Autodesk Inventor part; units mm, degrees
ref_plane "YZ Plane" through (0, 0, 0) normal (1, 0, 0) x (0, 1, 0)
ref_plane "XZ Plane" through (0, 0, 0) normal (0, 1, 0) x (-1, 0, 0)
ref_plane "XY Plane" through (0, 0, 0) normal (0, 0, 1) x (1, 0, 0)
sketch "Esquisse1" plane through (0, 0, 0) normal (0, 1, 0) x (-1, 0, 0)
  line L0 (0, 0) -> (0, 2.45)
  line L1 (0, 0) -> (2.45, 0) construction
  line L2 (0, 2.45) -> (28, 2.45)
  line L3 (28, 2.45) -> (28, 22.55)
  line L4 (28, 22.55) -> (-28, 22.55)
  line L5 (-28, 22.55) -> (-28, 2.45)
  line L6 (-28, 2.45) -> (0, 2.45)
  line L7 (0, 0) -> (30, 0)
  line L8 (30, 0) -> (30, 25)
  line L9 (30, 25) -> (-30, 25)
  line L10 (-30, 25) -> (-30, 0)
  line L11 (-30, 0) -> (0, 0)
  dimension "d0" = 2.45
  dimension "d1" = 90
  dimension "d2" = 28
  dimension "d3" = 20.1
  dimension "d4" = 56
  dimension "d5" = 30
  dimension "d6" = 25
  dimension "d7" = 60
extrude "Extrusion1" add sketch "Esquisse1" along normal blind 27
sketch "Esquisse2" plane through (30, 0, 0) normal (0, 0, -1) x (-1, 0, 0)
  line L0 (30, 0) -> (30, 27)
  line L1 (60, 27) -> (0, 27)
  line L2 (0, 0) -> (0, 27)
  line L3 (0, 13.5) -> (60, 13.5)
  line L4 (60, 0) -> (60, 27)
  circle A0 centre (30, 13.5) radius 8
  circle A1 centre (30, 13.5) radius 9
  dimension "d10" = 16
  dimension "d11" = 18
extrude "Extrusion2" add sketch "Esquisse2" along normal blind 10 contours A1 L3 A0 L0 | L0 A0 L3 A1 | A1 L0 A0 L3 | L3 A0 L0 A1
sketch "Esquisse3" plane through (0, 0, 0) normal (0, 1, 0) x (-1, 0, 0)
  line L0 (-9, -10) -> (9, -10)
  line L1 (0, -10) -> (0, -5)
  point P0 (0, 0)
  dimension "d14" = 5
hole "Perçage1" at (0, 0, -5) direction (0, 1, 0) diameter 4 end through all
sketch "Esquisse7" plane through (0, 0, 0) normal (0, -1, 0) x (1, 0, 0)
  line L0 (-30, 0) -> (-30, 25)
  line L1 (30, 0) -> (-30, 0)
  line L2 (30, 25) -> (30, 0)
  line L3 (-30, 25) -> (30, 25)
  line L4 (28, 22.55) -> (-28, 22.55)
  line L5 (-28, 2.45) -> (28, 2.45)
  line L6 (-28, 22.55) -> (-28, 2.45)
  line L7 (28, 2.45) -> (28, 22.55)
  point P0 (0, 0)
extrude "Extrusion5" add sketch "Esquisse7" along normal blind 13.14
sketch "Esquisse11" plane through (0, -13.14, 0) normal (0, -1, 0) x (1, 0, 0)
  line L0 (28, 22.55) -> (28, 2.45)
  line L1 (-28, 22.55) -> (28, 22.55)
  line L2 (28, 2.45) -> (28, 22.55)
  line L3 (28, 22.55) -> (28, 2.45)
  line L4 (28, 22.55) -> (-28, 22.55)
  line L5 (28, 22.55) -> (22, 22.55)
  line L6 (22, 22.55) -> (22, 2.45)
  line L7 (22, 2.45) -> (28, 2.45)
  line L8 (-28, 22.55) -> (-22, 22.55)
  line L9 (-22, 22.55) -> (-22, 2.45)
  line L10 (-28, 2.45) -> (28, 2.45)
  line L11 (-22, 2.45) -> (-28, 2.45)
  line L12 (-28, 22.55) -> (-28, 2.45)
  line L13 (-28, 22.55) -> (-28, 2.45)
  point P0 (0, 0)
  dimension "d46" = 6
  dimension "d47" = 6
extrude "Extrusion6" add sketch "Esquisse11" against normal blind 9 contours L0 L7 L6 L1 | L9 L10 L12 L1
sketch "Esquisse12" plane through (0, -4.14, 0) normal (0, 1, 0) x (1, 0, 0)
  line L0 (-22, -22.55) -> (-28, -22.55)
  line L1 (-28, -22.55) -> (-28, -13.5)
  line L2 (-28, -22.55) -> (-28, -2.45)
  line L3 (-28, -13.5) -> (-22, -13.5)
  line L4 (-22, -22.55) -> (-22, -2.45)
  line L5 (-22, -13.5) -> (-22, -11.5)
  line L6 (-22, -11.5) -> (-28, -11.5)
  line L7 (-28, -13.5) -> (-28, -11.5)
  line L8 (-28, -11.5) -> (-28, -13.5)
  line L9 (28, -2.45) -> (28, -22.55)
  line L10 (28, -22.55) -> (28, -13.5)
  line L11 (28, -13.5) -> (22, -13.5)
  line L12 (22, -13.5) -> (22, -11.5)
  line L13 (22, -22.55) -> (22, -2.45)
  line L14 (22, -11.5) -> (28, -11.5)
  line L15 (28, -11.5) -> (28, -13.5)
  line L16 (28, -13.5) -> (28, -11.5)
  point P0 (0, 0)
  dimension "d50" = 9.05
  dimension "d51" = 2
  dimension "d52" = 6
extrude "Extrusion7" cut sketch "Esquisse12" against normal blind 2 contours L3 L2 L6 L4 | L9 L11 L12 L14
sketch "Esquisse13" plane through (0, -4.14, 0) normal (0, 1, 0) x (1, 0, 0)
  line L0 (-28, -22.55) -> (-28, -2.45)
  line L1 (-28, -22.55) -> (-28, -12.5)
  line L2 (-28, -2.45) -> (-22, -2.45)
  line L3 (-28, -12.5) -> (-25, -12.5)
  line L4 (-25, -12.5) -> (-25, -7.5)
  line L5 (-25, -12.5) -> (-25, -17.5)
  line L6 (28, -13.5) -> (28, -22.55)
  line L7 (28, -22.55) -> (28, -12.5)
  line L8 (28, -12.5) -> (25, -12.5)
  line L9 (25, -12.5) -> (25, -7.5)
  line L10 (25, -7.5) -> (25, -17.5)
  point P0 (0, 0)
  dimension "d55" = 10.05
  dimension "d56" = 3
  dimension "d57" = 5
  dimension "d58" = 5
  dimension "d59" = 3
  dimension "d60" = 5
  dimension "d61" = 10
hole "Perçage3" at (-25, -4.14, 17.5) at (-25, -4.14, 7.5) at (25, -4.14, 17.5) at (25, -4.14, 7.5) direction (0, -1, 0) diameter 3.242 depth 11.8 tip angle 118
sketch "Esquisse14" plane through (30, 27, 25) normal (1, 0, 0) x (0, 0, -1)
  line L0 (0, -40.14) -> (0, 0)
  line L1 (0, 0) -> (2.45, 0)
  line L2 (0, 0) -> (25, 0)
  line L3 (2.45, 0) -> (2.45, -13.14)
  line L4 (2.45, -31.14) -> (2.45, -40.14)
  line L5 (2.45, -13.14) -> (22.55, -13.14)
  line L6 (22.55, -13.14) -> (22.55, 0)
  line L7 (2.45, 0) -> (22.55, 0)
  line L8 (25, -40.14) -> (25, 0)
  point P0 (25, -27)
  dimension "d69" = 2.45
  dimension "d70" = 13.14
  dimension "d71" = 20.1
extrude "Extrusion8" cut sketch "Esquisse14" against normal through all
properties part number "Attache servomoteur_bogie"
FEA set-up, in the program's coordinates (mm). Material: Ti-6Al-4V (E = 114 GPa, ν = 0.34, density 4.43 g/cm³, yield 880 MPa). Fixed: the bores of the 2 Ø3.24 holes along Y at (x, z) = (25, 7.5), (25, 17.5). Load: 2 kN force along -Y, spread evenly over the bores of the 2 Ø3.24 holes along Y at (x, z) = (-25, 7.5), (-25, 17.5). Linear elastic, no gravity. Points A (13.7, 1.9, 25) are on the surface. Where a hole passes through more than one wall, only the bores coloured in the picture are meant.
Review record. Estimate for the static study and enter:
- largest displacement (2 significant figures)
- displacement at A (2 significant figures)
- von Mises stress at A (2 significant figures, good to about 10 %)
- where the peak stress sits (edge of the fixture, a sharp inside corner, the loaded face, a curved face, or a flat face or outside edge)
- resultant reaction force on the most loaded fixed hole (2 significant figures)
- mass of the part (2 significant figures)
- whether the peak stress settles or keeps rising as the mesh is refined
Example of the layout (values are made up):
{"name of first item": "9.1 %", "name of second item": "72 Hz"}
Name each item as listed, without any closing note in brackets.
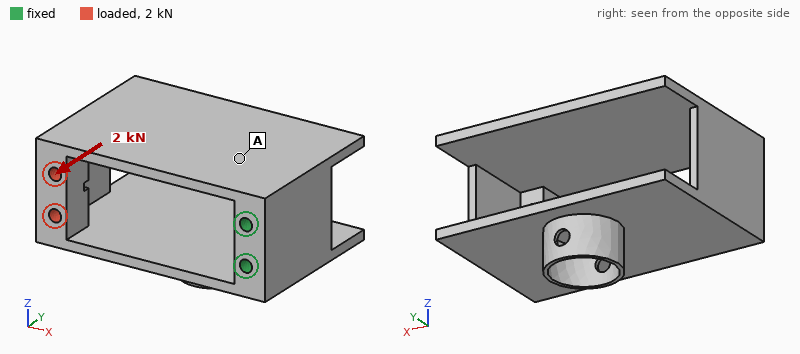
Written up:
{"largest displacement": "0.79 mm", "displacement at A": "0.18 mm", "von Mises stress at A": "67 MPa", "where the peak stress sits": "edge of the fixture", "resultant reaction force on the most loaded fixed hole": "1.0 kN", "mass of the part": "72 g", "whether the peak stress settles or keeps rising as the mesh is refined": "keeps rising"}
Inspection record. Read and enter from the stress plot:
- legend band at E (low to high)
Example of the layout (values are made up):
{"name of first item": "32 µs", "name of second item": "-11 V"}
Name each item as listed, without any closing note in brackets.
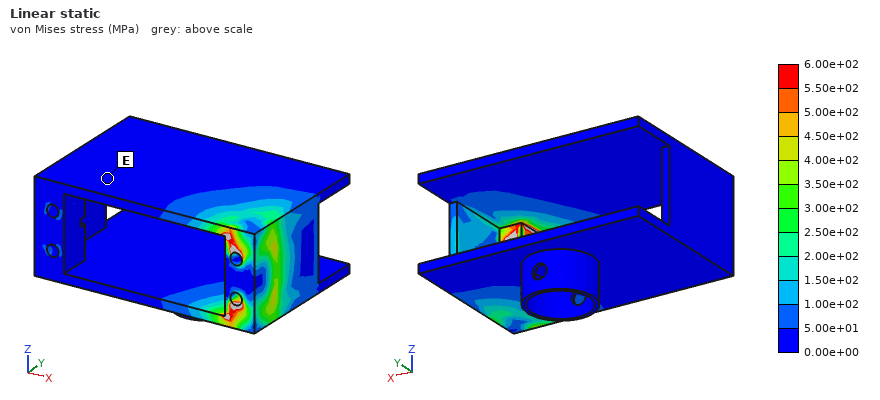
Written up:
{"legend band at E": "0.00e+00 to 5.00e+01 MPa"}
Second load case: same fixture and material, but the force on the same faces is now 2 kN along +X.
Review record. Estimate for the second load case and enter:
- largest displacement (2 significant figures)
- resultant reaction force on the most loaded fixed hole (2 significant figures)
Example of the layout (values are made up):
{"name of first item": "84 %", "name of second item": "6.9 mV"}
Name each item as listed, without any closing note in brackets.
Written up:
{"largest displacement": "41 µm", "resultant reaction force on the most loaded fixed hole": "1.1 kN"}
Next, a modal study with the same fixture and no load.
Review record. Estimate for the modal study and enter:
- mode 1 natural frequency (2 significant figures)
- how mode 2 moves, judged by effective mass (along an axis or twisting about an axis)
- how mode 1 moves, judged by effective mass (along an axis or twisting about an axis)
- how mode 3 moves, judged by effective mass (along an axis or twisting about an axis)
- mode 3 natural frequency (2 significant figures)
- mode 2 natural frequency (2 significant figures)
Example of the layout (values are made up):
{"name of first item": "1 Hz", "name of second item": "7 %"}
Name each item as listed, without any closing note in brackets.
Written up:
{"mode 1 natural frequency": "770 Hz", "how mode 2 moves, judged by effective mass": "along Y", "how mode 1 moves, judged by effective mass": "along Z", "how mode 3 moves, judged by effective mass": "twisting about X", "mode 3 natural frequency": "1900 Hz", "mode 2 natural frequency": "1500 Hz"}
